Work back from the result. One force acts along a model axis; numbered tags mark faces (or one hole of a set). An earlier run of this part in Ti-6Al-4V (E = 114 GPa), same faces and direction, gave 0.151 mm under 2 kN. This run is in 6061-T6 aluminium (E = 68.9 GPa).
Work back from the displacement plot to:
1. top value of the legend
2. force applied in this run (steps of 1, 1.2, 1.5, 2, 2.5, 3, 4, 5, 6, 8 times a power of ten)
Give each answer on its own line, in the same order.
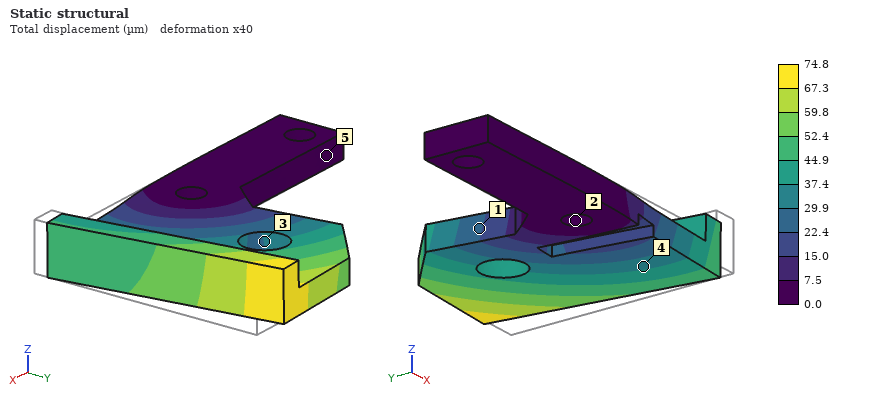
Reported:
74.8 µm
600 N
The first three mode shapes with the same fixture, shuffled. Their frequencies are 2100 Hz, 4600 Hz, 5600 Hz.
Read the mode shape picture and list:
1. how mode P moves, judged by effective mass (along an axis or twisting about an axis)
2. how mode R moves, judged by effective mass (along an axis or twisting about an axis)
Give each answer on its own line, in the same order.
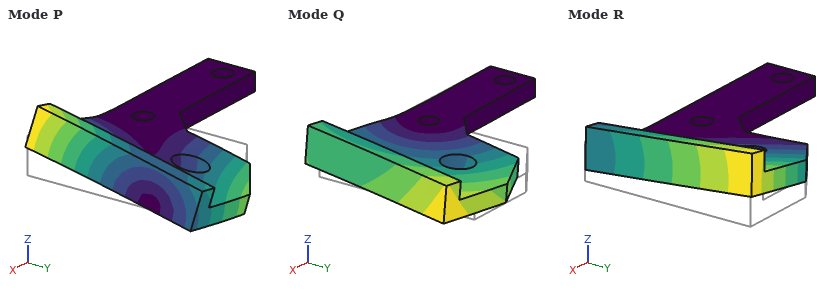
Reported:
twisting about X
along Z
